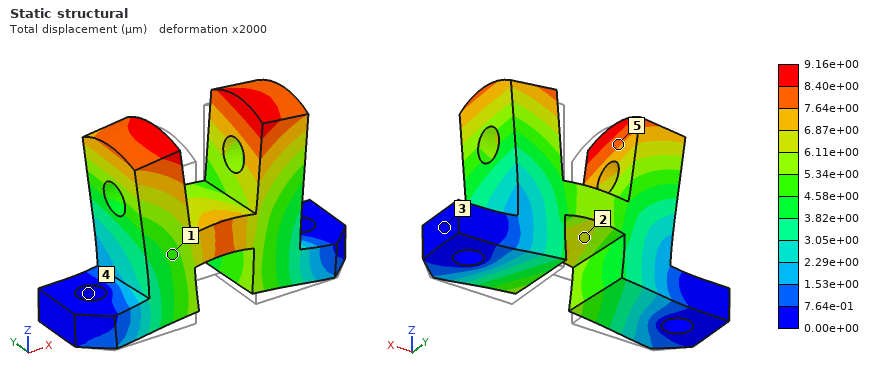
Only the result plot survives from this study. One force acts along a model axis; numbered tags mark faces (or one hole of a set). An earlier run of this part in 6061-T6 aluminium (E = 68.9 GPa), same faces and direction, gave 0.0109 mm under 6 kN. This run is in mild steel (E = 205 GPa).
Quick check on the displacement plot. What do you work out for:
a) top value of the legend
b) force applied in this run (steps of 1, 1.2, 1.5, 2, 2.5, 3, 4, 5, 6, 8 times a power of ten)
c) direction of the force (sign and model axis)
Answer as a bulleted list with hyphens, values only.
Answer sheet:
- 9.16e+00 µm
- 15 kN
- +Z
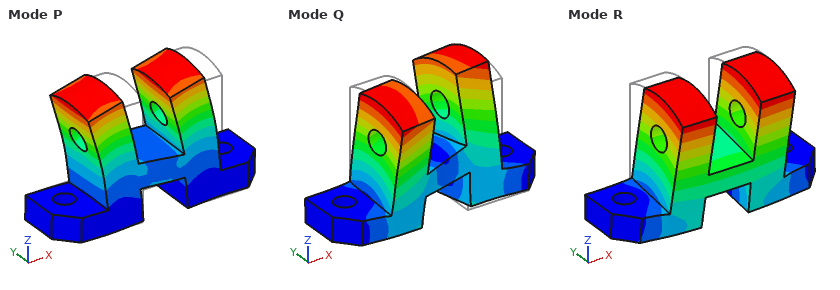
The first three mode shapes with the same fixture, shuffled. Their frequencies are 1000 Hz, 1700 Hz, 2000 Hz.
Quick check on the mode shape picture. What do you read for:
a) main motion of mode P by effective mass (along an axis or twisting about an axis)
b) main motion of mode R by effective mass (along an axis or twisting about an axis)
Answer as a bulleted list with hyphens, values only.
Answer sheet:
- along X
- along Y
